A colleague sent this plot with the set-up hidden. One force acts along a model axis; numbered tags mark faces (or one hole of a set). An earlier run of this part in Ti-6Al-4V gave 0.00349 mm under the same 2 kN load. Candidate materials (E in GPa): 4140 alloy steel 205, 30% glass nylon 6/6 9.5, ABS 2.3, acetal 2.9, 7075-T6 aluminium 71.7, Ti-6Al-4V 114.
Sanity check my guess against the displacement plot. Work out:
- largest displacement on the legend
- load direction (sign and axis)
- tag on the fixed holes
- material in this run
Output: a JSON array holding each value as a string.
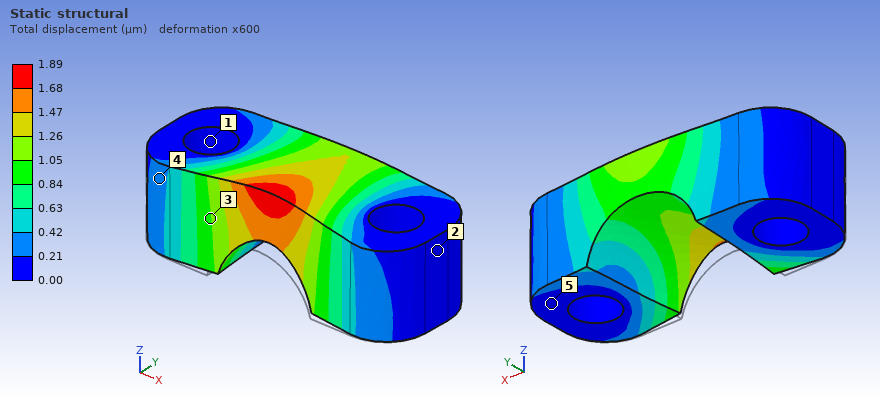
["1.89 µm", "+Y", "1", "4140 alloy steel"]
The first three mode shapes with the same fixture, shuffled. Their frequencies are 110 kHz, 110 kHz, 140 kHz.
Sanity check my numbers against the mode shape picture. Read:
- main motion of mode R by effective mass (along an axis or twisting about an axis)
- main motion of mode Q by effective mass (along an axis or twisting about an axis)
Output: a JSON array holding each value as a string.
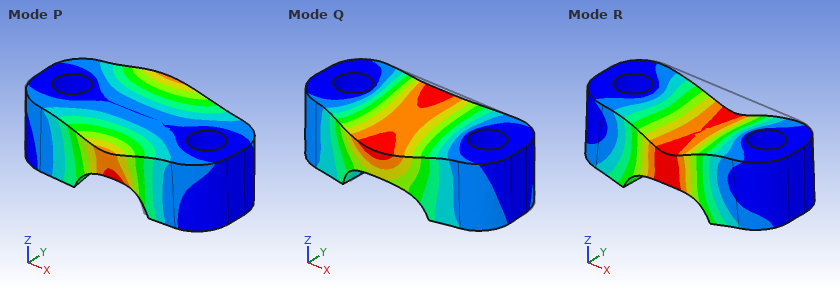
["along Z", "along Y"]
